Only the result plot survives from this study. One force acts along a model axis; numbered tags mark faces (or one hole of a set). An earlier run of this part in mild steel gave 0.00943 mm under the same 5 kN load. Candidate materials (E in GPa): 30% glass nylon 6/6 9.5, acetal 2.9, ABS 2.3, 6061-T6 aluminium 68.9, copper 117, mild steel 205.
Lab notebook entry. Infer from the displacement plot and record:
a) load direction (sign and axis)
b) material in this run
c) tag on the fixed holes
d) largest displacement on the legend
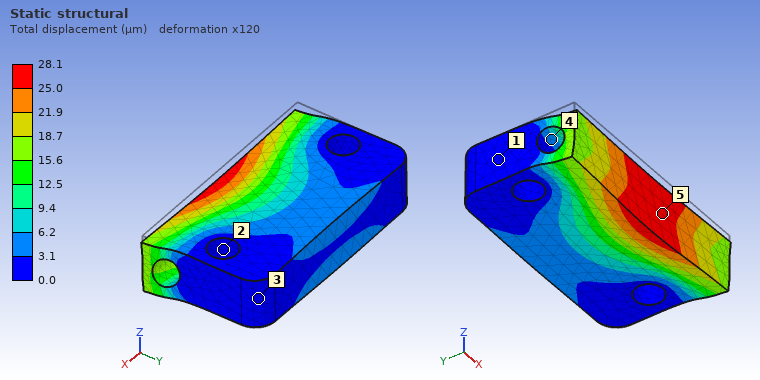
-Z
6061-T6 aluminium
2
28.1 µm
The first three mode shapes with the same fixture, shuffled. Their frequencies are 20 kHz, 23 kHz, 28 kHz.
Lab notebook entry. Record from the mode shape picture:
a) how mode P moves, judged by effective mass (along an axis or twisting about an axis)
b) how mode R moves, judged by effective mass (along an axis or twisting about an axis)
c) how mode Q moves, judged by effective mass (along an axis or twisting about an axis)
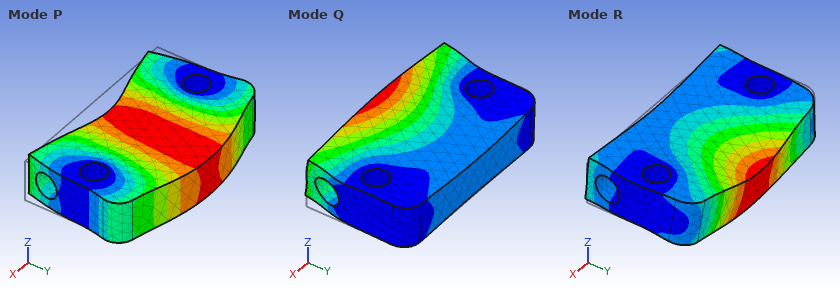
along Y
along Z
along Z
